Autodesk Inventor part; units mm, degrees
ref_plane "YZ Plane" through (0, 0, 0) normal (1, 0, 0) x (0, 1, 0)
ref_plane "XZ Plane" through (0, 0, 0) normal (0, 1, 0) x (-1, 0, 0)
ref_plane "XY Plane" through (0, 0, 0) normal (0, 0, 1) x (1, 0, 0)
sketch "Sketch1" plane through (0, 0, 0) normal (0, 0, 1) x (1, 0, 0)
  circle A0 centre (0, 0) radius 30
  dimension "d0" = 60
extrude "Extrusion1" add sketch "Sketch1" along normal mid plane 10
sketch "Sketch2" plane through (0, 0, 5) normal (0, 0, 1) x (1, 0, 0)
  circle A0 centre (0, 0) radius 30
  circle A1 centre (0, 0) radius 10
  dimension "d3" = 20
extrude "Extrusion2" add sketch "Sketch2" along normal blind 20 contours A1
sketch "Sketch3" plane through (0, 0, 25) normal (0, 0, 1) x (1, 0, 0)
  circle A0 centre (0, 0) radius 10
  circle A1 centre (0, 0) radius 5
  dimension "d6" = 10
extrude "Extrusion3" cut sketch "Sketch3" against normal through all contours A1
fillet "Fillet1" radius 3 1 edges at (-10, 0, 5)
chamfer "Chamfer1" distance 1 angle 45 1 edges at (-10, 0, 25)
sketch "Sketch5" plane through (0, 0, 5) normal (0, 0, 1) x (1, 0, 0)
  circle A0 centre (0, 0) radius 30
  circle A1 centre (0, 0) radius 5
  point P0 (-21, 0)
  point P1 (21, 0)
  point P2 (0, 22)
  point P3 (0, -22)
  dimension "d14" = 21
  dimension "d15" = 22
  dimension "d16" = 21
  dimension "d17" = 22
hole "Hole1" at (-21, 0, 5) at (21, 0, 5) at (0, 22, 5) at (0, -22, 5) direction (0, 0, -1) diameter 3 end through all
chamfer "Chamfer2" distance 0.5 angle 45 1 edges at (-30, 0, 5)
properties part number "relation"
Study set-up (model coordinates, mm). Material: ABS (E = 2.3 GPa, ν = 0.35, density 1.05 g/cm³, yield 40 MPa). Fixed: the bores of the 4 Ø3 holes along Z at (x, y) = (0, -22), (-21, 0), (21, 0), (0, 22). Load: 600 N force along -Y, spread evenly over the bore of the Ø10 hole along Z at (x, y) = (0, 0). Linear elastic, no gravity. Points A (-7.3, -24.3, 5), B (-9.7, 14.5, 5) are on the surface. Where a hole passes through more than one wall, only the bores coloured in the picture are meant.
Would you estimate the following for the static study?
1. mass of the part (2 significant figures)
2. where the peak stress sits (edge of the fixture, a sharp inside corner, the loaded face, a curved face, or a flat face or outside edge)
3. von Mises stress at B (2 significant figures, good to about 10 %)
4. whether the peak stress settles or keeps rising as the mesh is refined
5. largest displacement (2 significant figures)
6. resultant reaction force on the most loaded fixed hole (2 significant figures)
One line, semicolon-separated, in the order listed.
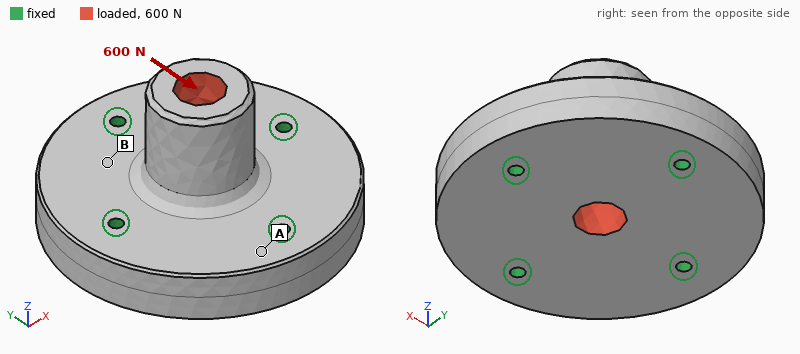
34 g; edge of the fixture; 1.2 MPa; keeps rising; 0.10 mm; 230 N
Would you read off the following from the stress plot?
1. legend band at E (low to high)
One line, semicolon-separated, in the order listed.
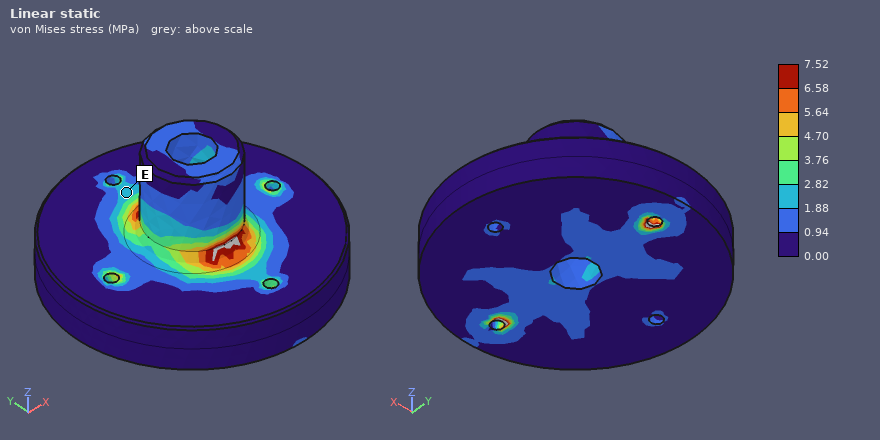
1.88 to 2.82 MPa
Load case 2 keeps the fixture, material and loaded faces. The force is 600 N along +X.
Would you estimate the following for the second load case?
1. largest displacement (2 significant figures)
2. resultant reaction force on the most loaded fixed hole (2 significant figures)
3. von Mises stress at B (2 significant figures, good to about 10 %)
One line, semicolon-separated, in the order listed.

99 µm; 250 N; 0.74 MPa
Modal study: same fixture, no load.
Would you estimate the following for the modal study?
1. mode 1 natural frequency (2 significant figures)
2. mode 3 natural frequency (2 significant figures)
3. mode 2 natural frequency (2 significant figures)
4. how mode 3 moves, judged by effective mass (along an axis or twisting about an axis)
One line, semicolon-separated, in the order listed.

5100 Hz; 6400 Hz; 5200 Hz; along Z
